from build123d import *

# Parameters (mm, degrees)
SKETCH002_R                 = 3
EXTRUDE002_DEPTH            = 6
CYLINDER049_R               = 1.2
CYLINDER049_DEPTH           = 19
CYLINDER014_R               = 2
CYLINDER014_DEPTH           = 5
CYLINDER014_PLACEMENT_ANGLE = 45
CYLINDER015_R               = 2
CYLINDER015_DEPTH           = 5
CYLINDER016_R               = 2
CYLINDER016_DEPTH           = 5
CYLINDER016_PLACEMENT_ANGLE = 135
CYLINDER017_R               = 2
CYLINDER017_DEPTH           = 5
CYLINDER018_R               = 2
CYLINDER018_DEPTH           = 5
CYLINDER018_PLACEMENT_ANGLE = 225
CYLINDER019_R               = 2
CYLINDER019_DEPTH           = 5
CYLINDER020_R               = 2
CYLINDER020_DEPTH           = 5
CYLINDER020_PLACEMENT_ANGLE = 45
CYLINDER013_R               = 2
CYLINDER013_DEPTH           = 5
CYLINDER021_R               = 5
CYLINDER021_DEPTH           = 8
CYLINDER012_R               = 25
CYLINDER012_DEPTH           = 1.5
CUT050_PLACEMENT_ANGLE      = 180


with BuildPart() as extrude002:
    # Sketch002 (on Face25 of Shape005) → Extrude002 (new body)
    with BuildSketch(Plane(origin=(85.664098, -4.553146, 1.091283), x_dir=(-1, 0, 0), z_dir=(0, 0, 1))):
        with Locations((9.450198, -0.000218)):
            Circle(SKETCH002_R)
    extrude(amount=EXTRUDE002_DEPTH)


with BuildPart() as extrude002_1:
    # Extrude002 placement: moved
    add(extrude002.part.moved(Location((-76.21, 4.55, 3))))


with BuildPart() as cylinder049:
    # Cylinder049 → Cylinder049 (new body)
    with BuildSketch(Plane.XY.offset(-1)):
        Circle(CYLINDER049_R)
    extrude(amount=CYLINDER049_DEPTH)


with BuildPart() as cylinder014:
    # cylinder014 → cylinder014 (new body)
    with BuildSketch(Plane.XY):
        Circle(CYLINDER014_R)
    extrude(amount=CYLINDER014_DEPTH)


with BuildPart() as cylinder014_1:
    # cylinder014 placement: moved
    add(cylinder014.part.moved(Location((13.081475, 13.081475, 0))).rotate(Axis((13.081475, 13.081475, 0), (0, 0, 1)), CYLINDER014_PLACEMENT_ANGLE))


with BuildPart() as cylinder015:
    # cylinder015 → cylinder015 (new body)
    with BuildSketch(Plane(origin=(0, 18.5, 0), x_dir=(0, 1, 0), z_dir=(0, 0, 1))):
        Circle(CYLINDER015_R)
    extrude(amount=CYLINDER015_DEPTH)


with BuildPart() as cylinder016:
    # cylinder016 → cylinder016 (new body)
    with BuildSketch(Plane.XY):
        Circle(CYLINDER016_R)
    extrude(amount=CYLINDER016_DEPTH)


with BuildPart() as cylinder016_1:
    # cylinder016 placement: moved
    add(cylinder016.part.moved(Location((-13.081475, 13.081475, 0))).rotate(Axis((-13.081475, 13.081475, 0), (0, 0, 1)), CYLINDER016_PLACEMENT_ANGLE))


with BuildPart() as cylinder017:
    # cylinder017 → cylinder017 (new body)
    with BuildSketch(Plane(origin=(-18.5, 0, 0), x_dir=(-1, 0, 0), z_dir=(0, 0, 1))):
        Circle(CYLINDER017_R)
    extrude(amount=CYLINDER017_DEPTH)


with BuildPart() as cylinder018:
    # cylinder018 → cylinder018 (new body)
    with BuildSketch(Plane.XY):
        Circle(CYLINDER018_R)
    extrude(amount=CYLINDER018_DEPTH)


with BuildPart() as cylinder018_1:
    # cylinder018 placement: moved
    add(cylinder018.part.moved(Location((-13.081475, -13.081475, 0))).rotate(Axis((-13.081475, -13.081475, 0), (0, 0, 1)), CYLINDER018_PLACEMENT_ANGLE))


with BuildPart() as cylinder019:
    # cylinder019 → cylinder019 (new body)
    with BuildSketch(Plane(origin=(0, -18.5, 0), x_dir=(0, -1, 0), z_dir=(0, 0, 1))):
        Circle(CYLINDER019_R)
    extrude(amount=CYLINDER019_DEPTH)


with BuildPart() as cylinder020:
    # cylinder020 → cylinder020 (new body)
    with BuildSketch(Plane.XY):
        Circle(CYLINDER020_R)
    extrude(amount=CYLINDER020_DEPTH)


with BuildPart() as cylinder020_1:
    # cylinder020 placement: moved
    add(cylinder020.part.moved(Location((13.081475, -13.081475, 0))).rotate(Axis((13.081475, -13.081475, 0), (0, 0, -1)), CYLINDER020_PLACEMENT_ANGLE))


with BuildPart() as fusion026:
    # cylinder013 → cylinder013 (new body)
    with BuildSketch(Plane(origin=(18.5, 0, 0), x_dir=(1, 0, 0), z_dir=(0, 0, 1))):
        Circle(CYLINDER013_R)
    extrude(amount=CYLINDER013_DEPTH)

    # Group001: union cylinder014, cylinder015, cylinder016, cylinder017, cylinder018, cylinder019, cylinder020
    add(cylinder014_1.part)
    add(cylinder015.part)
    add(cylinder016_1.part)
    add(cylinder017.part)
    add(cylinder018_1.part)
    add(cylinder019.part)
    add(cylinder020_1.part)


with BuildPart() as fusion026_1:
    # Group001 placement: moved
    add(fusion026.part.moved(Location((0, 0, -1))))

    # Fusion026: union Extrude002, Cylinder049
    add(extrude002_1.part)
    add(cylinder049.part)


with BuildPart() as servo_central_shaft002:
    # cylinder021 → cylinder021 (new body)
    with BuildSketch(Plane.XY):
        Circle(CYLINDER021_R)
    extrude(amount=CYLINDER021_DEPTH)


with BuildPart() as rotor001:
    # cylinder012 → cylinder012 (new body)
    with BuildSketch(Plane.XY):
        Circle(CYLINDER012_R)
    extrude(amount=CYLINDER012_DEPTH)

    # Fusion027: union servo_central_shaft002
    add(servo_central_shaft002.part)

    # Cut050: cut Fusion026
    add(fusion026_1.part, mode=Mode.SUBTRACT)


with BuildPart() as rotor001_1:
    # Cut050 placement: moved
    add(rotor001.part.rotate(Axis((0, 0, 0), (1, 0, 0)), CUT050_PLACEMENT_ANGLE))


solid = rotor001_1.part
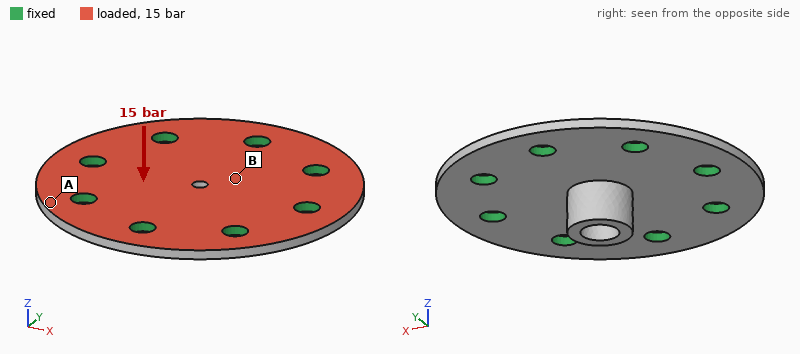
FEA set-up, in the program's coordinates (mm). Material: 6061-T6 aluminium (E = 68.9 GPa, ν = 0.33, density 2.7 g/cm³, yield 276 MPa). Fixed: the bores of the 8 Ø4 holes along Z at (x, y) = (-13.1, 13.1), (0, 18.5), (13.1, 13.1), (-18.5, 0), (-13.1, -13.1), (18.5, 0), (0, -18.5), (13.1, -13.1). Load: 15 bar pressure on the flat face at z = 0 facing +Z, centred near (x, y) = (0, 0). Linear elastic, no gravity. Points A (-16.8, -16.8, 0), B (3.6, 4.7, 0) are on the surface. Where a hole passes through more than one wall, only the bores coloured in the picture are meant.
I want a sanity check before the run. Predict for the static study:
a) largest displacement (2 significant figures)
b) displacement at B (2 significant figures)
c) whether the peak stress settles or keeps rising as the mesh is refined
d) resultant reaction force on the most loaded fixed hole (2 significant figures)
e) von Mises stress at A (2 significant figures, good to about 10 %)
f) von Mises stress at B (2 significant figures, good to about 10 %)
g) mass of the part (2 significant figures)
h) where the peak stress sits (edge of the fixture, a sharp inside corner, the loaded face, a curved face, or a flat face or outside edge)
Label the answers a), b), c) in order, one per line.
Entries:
a) 70 µm
b) 67 µm
c) keeps rising
d) 350 N
e) 28 MPa
f) 82 MPa
g) 8.6 g
h) edge of the fixture
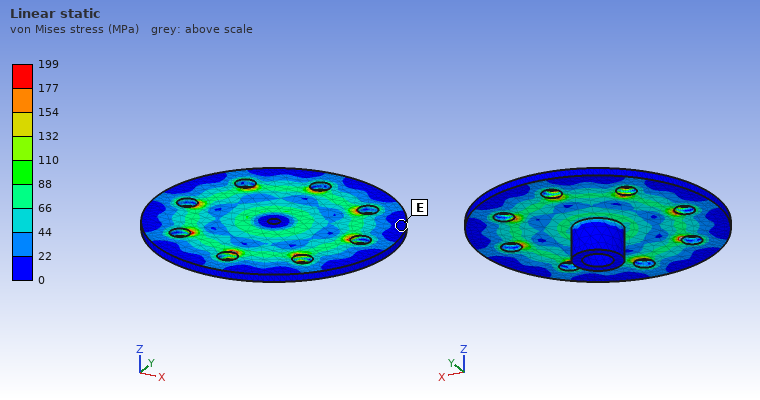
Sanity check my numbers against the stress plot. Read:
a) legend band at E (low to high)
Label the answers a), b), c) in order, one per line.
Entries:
a) 0 to 22 MPa
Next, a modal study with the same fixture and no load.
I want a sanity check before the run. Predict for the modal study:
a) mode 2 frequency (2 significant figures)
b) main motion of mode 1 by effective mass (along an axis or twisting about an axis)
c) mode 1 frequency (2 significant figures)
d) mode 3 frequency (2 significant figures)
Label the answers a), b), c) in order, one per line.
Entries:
a) 17 kHz
b) along Z
c) 9600 Hz
d) 17 kHz
